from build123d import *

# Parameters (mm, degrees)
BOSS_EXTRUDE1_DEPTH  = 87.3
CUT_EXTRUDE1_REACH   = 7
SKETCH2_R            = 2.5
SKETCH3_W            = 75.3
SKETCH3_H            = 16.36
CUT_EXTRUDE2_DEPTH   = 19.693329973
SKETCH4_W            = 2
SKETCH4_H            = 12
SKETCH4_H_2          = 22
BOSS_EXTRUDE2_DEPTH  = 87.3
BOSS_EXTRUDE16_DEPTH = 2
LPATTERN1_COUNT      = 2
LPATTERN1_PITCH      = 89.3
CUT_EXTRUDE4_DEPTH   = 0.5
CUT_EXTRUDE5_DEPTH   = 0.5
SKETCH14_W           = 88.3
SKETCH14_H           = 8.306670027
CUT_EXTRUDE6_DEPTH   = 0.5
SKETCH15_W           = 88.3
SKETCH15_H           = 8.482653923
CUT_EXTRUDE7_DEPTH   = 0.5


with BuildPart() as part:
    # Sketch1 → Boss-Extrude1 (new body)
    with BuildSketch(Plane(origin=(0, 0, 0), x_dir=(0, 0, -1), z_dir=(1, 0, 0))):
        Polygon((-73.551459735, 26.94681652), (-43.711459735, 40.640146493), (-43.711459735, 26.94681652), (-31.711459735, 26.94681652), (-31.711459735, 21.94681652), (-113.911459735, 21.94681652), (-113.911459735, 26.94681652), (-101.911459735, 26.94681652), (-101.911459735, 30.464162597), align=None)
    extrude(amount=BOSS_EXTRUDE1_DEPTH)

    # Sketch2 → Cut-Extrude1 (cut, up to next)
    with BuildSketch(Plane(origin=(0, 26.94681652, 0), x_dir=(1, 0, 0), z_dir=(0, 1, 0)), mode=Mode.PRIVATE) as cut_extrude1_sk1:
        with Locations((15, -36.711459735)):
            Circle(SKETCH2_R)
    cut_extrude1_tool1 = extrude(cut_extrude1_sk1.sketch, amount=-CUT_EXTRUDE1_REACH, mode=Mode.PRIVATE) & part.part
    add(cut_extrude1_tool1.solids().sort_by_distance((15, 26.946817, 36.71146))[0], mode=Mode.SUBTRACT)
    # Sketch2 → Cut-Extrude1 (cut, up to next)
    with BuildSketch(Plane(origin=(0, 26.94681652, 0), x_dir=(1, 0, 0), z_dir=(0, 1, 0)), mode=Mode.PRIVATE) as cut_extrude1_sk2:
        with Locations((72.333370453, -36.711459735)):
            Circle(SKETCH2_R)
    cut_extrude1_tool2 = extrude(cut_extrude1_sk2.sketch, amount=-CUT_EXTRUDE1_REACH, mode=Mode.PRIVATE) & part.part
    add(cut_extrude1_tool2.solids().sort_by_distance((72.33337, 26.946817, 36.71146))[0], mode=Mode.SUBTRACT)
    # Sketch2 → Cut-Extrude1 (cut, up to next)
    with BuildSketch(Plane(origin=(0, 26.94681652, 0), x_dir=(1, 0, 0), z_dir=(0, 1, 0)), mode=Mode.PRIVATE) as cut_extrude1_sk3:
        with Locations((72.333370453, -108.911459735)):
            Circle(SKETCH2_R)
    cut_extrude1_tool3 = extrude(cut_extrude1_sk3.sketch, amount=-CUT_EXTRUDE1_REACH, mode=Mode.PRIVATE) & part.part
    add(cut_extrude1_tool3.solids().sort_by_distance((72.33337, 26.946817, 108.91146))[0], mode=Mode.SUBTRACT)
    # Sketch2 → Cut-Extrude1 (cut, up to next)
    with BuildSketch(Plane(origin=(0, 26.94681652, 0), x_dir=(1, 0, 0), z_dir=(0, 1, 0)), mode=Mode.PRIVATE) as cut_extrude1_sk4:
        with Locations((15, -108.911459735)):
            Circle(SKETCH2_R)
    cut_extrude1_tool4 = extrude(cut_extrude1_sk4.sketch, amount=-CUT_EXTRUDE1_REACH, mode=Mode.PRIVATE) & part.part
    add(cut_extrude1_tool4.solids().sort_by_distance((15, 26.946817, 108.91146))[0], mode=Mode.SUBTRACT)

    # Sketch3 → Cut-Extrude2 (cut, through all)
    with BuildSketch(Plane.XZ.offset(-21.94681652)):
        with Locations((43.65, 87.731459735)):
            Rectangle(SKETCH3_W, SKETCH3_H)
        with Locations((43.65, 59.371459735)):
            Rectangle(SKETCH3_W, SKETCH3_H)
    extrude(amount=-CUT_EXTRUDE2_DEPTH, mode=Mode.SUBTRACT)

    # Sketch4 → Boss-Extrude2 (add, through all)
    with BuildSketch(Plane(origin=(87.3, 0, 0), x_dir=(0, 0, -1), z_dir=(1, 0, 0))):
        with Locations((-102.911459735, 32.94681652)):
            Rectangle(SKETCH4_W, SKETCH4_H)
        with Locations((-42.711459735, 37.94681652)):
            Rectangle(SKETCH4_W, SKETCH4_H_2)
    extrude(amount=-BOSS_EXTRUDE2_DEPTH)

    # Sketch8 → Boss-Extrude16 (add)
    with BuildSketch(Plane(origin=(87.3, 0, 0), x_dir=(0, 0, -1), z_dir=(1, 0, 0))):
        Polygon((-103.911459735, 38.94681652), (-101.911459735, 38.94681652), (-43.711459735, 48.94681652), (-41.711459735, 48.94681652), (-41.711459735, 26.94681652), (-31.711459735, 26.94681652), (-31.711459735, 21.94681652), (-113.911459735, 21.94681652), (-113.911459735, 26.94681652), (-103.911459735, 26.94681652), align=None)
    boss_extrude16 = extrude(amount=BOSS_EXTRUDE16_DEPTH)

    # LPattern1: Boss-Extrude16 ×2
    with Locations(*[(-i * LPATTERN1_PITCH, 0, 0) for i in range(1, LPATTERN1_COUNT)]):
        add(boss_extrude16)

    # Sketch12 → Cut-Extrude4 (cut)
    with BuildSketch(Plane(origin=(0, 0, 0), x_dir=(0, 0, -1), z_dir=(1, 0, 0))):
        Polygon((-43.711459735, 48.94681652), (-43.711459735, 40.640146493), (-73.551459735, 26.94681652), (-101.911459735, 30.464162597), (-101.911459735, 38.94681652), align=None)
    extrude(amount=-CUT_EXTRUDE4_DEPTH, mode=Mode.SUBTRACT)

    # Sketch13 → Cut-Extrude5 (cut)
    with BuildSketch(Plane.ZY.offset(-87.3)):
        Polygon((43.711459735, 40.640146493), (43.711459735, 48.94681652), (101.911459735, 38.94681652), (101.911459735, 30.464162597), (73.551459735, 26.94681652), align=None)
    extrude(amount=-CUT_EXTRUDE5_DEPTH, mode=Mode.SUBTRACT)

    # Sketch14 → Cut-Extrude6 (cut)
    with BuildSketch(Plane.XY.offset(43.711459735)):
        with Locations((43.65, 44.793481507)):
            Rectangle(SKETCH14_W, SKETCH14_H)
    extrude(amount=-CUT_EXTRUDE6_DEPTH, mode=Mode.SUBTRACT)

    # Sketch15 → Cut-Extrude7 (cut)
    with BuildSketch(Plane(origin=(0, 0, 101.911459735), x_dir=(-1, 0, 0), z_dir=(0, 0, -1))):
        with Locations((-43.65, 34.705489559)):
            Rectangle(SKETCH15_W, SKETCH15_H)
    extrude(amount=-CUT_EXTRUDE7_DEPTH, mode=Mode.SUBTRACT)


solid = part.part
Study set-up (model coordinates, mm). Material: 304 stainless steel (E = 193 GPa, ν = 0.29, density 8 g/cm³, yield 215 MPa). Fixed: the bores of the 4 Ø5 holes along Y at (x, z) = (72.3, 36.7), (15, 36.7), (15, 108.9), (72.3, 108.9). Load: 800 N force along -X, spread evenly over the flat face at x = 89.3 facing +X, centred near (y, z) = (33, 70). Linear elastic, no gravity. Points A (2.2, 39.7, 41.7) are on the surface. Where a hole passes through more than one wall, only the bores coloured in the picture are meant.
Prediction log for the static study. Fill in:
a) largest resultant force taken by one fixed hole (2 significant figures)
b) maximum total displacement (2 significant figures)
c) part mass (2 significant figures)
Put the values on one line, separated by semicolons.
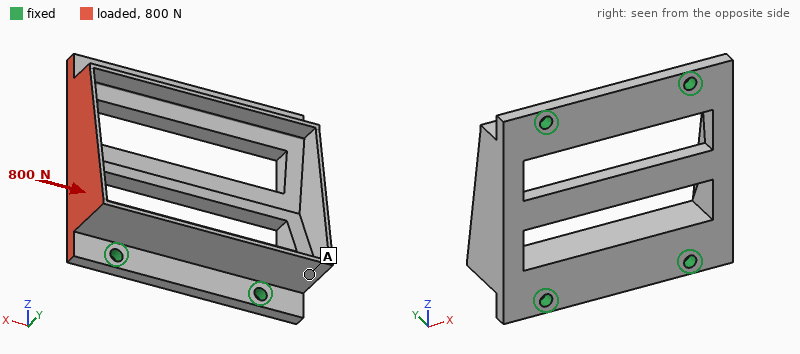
260 N; 48 µm; 360 g
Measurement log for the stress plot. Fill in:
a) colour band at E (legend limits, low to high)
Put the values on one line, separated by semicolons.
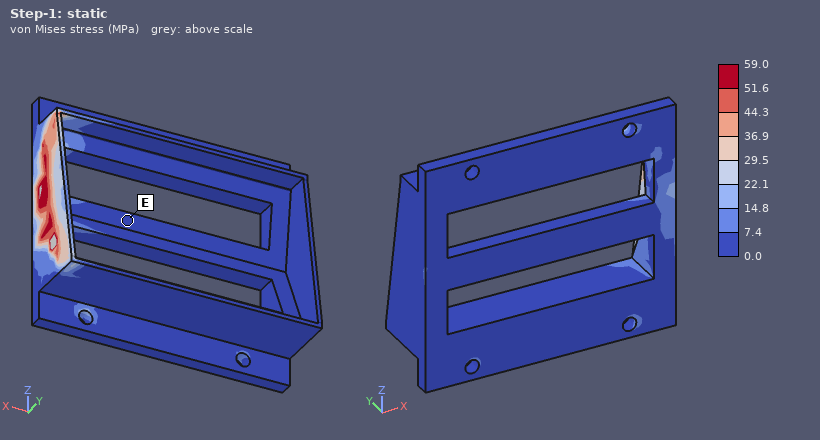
0.0 to 7.4 MPa
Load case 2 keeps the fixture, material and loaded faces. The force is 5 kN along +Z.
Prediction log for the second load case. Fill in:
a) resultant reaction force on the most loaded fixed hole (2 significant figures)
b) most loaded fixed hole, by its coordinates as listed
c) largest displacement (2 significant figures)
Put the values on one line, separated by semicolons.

3.3 kN; (72.3, 36.7); 22 µm
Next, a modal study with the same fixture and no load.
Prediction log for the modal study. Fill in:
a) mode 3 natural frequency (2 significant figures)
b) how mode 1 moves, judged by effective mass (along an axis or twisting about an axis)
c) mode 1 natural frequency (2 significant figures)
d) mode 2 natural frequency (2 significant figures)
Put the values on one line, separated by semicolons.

6000 Hz; along Y; 3200 Hz; 5800 Hz
